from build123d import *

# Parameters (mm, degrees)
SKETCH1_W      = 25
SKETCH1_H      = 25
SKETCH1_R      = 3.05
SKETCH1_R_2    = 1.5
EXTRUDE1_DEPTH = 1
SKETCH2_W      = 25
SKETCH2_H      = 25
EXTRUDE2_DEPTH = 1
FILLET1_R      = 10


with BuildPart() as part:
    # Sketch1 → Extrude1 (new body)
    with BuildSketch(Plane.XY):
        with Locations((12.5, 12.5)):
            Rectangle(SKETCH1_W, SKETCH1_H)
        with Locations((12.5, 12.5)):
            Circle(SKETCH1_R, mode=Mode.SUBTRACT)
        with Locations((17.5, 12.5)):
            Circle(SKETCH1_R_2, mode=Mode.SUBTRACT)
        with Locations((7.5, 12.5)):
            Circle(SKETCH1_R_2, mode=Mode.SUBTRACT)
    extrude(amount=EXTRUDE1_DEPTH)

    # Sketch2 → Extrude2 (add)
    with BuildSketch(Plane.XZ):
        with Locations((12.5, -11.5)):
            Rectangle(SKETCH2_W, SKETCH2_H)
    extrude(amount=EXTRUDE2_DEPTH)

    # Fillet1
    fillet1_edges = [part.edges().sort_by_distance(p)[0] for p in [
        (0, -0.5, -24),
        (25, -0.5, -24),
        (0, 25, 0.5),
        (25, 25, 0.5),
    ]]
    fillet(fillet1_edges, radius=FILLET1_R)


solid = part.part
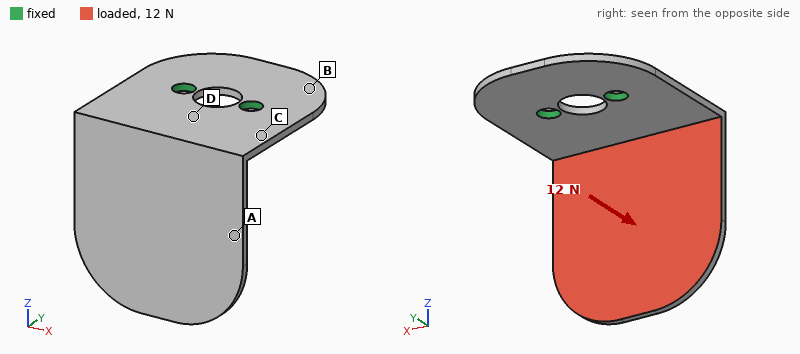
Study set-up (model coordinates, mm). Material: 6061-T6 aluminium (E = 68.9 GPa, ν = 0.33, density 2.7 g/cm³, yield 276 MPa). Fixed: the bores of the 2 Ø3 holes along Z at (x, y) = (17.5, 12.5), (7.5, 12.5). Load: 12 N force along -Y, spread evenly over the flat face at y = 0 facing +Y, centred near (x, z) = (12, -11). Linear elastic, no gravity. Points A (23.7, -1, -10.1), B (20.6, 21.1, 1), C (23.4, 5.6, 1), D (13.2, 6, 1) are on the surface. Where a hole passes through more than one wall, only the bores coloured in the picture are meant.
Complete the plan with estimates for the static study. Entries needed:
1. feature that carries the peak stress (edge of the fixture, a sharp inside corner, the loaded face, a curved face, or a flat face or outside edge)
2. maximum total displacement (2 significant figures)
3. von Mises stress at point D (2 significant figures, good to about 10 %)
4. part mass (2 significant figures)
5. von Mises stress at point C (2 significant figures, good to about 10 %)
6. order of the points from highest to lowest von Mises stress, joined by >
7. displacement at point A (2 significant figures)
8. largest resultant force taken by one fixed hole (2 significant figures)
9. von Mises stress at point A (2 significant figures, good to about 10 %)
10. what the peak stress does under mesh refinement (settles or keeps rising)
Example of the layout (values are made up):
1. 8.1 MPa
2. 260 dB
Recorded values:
1. edge of the fixture
2. 0.43 mm
3. 27 MPa
4. 3.0 g
5. 33 MPa
6. C > D > A > B
7. 0.18 mm
8. 6.3 N
9. 10 MPa
10. keeps rising
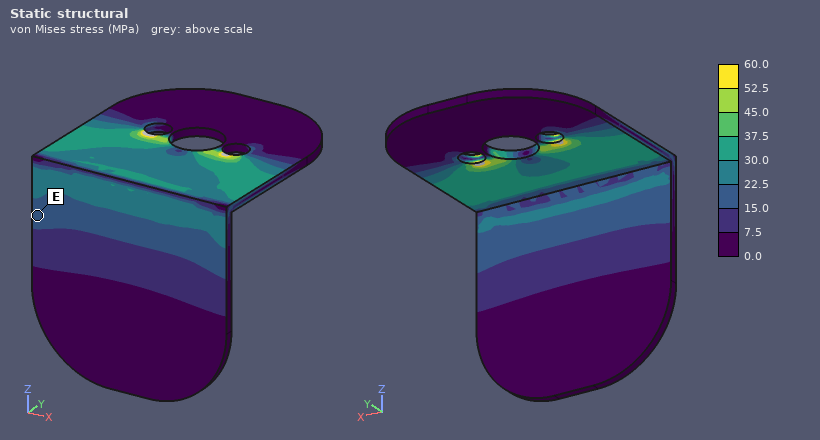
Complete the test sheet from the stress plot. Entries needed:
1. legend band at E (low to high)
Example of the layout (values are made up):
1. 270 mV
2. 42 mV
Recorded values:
1. 15.0 to 22.5 MPa
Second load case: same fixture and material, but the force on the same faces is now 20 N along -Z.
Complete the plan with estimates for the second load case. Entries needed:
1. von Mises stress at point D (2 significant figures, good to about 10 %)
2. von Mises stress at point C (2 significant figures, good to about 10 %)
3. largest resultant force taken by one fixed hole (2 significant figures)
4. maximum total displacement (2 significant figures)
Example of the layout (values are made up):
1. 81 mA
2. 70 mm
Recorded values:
1. 23 MPa
2. 27 MPa
3. 10 N
4. 0.25 mm
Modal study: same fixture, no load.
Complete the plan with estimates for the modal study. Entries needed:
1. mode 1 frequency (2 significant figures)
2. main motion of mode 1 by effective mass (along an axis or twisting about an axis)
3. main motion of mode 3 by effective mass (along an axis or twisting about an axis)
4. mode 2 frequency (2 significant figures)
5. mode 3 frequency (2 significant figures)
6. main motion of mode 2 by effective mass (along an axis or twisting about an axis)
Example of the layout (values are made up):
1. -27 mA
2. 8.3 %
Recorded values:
1. 830 Hz
2. along Y
3. along Z
4. 1600 Hz
5. 2700 Hz
6. along X
